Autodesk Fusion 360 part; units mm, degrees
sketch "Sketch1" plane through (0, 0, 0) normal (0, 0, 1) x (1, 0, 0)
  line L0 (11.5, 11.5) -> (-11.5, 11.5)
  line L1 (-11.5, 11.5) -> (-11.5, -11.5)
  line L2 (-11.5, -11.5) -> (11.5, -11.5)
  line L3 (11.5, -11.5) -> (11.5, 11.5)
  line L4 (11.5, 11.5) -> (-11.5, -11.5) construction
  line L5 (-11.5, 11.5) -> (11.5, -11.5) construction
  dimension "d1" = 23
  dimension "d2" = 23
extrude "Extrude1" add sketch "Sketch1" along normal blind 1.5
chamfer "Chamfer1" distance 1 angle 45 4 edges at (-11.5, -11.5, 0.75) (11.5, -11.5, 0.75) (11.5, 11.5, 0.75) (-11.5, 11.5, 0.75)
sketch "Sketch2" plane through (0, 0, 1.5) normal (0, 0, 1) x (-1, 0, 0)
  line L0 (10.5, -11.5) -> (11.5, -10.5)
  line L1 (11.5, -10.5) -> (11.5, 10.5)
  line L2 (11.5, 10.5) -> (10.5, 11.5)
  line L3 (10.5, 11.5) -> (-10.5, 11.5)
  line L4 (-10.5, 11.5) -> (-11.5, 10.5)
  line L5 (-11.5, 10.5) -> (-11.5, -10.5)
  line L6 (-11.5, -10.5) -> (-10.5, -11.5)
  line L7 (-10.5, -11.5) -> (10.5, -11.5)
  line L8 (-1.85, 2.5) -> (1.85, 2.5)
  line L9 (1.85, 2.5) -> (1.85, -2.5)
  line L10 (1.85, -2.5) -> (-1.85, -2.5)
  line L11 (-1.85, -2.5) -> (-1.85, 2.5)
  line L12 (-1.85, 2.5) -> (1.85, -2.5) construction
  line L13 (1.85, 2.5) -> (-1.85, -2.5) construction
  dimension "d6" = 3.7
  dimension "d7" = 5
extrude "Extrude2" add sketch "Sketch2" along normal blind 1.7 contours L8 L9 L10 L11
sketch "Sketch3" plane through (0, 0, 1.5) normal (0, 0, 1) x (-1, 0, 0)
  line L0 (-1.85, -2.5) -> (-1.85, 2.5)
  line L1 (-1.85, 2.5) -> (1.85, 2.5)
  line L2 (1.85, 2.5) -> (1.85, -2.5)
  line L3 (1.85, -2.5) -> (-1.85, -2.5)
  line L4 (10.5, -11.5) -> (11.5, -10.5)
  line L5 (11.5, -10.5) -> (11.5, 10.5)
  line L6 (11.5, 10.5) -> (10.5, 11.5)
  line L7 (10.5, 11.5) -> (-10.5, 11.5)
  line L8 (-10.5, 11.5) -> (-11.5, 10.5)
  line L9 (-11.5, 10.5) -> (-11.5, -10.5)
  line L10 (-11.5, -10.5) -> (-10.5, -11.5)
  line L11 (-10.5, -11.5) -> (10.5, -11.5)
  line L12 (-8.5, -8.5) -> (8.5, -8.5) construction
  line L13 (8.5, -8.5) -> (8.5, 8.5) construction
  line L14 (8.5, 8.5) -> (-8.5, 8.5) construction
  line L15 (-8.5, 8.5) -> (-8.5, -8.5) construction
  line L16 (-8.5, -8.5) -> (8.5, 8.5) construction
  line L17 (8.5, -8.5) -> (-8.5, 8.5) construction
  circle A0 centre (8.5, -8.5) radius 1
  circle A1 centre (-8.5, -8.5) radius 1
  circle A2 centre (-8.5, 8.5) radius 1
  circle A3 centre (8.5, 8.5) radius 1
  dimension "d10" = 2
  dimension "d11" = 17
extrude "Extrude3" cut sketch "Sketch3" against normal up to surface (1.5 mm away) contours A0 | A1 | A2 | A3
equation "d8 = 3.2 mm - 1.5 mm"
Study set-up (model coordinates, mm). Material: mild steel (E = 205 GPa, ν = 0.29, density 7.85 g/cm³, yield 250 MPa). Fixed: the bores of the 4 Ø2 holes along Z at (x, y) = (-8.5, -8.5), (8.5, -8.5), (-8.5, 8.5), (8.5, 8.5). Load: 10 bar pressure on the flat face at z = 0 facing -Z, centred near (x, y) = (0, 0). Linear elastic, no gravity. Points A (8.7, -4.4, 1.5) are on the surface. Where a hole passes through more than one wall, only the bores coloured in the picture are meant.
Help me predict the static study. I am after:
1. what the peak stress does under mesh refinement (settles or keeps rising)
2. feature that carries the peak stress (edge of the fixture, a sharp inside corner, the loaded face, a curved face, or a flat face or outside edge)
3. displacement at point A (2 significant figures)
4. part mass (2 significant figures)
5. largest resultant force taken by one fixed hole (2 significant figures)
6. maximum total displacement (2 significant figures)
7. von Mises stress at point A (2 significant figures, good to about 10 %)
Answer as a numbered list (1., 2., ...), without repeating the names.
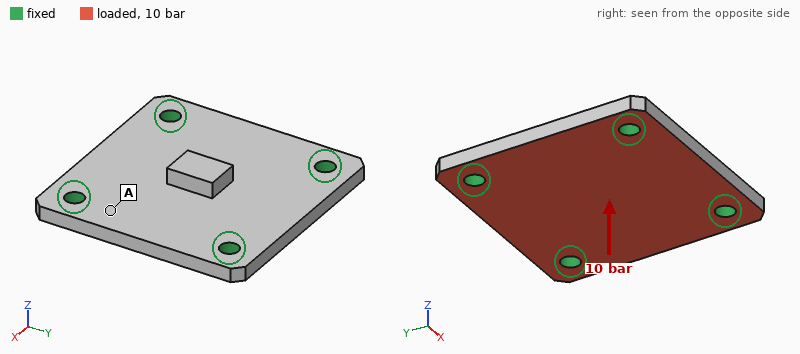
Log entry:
1. keeps rising
2. edge of the fixture
3. 2.3 µm
4. 6.3 g
5. 130 N
6. 7.1 µm
7. 18 MPa
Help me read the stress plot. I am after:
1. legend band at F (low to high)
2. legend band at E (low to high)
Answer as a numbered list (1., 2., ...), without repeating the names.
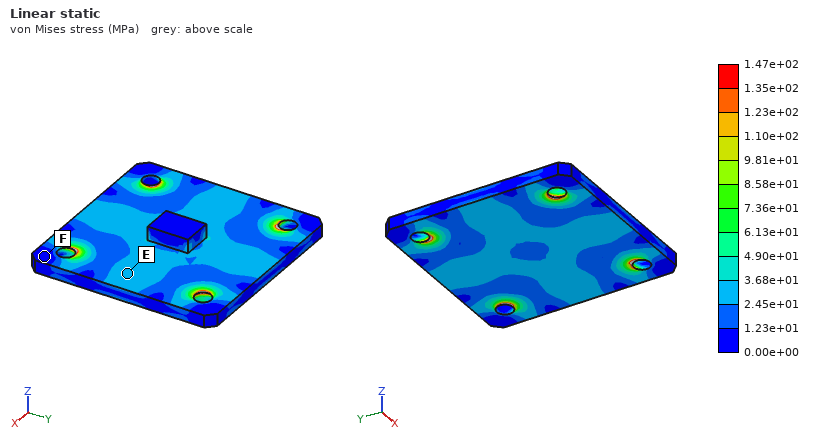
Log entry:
1. 0.00e+00 to 1.23e+01 MPa
2. 2.45e+01 to 3.68e+01 MPa
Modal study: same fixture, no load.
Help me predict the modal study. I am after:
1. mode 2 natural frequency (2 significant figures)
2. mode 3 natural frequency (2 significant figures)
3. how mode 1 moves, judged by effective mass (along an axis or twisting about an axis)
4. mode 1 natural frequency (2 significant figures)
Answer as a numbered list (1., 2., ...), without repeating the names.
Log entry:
1. 31 kHz
2. 31 kHz
3. along Z
4. 19 kHz
